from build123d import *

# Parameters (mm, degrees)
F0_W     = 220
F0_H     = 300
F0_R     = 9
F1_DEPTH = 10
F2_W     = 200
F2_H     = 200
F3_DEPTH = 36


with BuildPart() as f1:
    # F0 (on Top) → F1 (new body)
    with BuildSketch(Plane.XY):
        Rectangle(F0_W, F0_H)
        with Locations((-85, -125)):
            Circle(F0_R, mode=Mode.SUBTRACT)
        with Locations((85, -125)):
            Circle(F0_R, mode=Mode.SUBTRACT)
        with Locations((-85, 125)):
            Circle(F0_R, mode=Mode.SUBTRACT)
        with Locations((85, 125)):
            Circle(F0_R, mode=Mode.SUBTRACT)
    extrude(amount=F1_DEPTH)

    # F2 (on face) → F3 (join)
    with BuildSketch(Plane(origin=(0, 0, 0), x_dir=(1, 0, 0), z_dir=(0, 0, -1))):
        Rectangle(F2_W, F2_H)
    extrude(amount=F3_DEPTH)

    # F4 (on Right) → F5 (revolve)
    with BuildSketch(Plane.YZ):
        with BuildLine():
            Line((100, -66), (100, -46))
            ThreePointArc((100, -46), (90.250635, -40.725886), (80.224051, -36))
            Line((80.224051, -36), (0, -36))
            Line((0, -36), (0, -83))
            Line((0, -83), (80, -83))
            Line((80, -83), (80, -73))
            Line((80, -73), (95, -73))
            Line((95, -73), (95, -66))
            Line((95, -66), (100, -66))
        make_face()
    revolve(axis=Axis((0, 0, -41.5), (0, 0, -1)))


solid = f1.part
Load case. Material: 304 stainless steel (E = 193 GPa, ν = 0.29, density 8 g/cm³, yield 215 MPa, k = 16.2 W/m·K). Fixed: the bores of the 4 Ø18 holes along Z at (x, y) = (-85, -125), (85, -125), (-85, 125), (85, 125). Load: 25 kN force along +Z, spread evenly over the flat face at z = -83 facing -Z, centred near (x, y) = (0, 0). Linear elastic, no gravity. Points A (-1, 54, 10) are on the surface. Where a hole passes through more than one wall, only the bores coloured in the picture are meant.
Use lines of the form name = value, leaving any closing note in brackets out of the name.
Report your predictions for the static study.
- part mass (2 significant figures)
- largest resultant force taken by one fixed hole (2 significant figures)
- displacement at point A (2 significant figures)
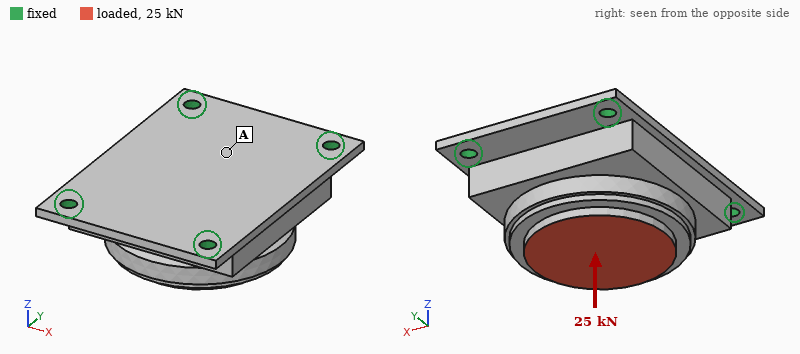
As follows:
part mass = 27 kg
largest resultant force taken by one fixed hole = 8.1 kN
displacement at point A = 21 µm
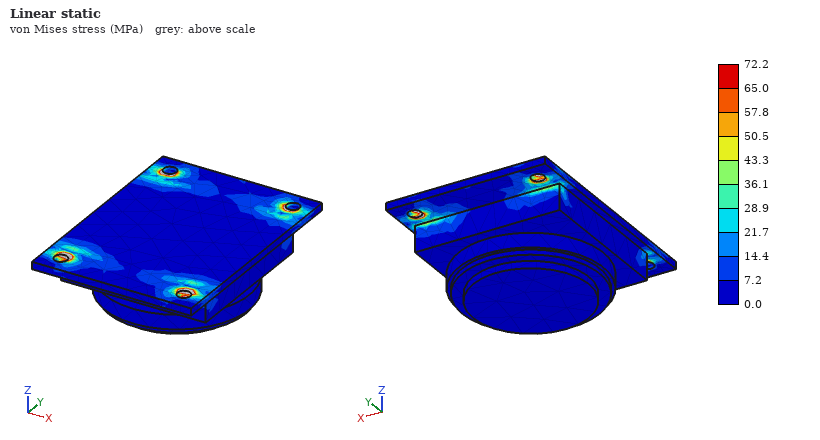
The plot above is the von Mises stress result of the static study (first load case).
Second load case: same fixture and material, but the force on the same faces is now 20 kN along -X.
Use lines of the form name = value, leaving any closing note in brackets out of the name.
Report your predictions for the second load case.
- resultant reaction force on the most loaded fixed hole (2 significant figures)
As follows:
resultant reaction force on the most loaded fixed hole = 8.9 kN
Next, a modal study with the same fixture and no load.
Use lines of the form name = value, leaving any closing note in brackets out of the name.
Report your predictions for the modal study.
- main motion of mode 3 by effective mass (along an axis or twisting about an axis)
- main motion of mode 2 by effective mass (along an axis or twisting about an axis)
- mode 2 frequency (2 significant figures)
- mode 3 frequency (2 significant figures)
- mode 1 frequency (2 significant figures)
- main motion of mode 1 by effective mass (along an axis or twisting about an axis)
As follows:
main motion of mode 3 by effective mass = along Y
main motion of mode 2 by effective mass = along X
mode 2 frequency = 1300 Hz
mode 3 frequency = 1700 Hz
mode 1 frequency = 1100 Hz
main motion of mode 1 by effective mass = along Z
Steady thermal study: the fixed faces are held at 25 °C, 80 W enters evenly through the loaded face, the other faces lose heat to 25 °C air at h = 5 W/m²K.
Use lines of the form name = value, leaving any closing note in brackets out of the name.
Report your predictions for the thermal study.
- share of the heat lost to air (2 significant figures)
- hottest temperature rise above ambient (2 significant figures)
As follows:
share of the heat lost to air = 44 %
hottest temperature rise above ambient = 58 K
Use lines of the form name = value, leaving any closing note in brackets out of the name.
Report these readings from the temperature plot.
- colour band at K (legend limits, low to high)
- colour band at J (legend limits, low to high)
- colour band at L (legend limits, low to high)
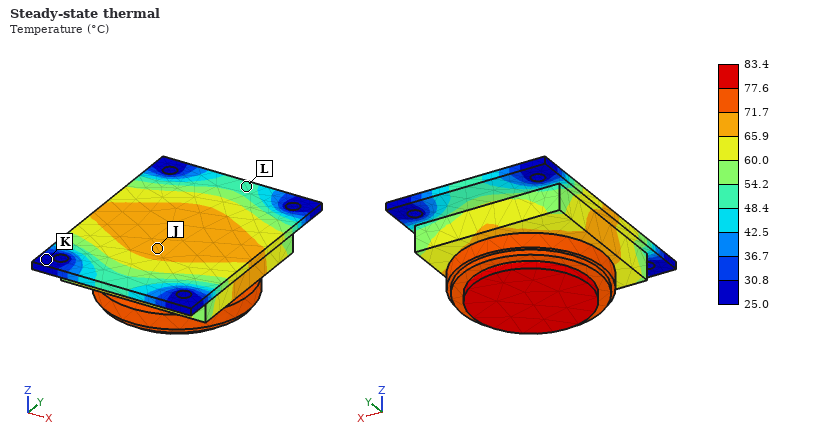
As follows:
colour band at K = 25.0 to 30.8 °C
colour band at J = 65.9 to 71.7 °C
colour band at L = 48.4 to 54.2 °C
